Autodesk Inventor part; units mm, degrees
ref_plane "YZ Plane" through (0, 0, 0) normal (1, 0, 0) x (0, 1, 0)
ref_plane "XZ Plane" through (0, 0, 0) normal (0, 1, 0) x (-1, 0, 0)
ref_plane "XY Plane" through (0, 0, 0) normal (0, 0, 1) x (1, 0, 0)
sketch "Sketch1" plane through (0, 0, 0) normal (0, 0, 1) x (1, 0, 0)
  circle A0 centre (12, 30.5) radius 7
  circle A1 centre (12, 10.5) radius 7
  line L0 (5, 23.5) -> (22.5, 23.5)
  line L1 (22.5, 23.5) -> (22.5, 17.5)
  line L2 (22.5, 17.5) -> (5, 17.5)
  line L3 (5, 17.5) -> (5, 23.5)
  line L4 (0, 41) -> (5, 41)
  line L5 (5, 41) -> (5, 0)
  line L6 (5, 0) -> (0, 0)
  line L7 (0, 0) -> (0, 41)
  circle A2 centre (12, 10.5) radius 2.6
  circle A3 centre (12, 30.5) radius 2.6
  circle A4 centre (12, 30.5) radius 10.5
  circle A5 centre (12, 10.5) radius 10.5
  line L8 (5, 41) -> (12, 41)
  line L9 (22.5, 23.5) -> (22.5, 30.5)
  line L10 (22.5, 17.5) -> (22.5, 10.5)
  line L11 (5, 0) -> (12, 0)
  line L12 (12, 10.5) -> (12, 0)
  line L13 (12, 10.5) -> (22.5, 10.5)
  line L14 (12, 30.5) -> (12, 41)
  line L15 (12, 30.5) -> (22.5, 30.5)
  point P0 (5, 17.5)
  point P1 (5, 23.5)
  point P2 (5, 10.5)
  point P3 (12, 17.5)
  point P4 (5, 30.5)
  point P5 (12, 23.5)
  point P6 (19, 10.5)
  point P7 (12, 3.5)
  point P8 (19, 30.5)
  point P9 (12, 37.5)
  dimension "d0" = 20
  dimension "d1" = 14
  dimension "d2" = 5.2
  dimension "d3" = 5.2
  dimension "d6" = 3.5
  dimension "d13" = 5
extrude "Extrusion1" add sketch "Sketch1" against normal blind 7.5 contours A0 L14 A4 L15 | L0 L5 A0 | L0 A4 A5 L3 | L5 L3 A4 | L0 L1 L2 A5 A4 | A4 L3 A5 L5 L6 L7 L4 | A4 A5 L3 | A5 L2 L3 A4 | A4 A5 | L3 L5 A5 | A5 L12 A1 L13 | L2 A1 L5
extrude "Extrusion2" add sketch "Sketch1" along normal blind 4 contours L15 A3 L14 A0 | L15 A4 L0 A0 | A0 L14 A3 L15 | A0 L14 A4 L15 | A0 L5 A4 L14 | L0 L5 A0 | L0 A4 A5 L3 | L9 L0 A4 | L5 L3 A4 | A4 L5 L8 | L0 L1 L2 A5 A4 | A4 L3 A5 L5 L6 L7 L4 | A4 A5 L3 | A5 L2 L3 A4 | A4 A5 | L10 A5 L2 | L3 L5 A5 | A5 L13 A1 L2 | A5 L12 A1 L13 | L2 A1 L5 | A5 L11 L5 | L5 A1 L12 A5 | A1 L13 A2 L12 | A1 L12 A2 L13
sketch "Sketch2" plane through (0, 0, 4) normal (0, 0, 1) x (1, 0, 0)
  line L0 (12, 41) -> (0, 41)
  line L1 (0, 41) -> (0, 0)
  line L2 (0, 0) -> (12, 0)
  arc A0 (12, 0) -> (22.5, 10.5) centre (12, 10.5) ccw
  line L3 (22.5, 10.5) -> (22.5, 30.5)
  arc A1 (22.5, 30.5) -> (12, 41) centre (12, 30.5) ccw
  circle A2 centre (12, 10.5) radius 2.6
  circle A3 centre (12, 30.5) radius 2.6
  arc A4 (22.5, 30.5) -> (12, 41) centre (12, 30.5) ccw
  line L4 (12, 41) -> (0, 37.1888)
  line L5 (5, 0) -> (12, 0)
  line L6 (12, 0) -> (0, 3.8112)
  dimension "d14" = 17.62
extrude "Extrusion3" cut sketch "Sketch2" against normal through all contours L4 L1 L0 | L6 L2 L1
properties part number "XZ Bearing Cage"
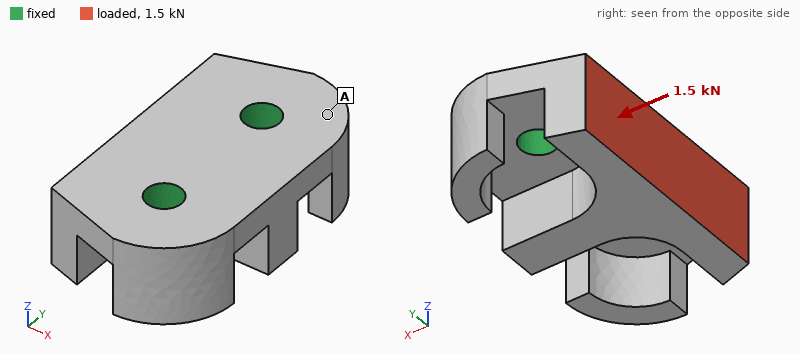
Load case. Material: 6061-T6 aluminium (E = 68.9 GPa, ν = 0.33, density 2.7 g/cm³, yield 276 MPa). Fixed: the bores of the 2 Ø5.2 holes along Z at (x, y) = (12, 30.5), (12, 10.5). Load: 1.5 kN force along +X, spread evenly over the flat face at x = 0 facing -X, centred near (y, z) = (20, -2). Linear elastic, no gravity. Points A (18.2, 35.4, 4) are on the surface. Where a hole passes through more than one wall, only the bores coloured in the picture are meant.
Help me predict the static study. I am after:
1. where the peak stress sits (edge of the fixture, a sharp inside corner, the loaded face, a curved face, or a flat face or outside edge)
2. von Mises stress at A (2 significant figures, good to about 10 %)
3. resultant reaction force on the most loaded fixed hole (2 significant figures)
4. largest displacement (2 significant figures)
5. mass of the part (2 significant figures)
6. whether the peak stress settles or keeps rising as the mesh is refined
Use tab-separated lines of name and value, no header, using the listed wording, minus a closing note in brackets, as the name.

where the peak stress sits	edge of the fixture
von Mises stress at A	7.4 MPa
resultant reaction force on the most loaded fixed hole	750 N
largest displacement	21 µm
mass of the part	17 g
whether the peak stress settles or keeps rising as the mesh is refined	keeps rising
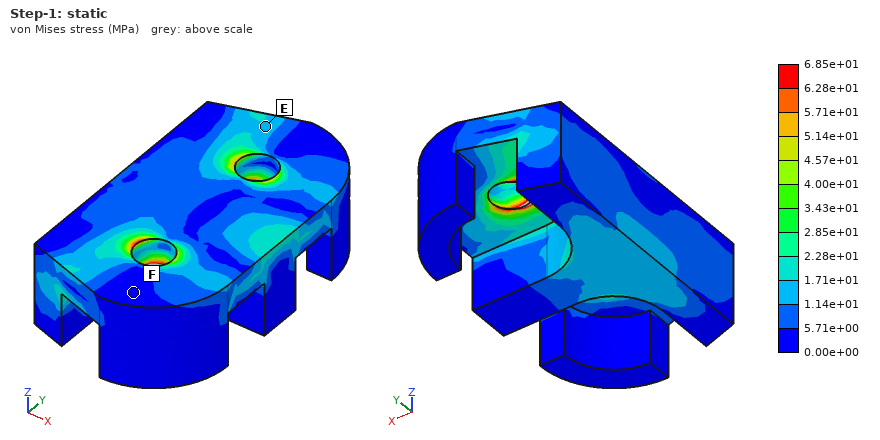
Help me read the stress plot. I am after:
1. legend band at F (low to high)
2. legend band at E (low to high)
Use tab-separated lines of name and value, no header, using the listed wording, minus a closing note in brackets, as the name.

legend band at F	0.00e+00 to 5.71e+00 MPa
legend band at E	1.14e+01 to 1.71e+01 MPa
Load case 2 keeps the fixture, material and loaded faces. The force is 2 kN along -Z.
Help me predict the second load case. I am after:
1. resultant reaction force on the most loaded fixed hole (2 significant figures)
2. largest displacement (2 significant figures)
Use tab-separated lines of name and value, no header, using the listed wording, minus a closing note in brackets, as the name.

resultant reaction force on the most loaded fixed hole	1.0 kN
largest displacement	64 µm
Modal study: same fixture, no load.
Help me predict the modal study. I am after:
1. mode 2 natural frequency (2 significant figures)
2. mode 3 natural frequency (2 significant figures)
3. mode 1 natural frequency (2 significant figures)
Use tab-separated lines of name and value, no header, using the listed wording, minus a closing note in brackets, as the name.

mode 2 natural frequency	18 kHz
mode 3 natural frequency	19 kHz
mode 1 natural frequency	14 kHz
